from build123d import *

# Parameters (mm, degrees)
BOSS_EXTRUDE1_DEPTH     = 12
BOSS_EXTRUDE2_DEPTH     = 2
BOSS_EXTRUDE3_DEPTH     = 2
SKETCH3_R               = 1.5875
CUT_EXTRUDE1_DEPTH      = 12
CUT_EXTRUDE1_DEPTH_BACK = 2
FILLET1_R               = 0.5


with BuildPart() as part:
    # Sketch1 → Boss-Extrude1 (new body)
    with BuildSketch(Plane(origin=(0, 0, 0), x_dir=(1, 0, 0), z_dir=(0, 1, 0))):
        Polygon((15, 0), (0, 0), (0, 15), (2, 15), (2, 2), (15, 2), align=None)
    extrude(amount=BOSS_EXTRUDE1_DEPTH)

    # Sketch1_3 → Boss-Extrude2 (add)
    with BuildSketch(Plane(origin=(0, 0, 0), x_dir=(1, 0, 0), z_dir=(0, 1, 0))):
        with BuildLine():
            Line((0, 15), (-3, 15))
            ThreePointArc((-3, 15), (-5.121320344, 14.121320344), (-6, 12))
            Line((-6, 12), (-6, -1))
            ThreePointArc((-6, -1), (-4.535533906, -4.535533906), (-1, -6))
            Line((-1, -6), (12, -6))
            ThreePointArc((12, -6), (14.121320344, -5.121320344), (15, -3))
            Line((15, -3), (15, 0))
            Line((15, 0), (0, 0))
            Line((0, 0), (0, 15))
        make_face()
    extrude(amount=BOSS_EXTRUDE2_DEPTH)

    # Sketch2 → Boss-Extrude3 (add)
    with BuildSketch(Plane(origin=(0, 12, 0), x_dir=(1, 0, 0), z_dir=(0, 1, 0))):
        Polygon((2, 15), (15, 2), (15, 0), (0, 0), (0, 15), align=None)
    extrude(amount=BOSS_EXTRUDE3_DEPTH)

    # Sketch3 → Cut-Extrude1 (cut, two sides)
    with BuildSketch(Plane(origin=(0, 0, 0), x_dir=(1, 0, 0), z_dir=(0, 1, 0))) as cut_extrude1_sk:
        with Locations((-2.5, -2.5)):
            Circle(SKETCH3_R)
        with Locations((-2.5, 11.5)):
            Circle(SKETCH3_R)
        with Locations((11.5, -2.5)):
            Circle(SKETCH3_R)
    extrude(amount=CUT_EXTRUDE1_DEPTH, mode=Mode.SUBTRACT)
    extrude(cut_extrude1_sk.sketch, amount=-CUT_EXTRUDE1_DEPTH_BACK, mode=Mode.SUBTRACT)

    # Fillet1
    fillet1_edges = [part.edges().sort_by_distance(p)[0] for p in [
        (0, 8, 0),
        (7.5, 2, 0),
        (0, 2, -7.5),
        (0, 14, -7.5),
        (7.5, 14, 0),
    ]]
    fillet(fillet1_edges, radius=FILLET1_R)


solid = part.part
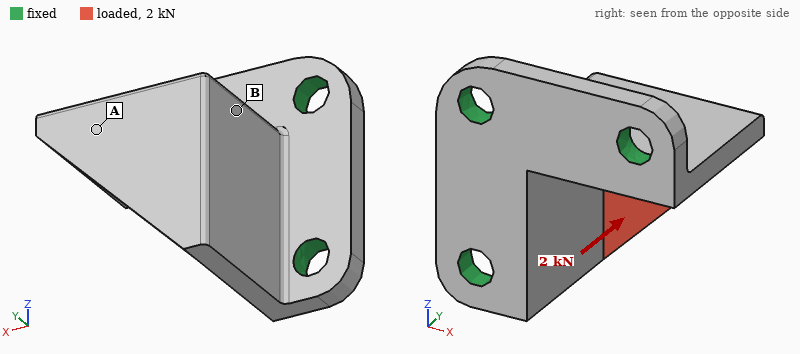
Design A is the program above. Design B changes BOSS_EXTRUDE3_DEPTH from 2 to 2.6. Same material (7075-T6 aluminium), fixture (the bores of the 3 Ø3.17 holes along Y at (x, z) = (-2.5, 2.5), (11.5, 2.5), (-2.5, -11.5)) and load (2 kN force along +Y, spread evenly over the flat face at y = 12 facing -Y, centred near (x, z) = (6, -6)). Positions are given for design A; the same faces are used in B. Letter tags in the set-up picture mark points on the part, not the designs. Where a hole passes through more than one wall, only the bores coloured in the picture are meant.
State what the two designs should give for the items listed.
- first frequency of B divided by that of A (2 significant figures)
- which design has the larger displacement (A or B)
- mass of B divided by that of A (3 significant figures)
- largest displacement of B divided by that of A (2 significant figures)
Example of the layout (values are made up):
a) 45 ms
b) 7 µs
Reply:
a) 0.96
b) A
c) 1.06
d) 0.79
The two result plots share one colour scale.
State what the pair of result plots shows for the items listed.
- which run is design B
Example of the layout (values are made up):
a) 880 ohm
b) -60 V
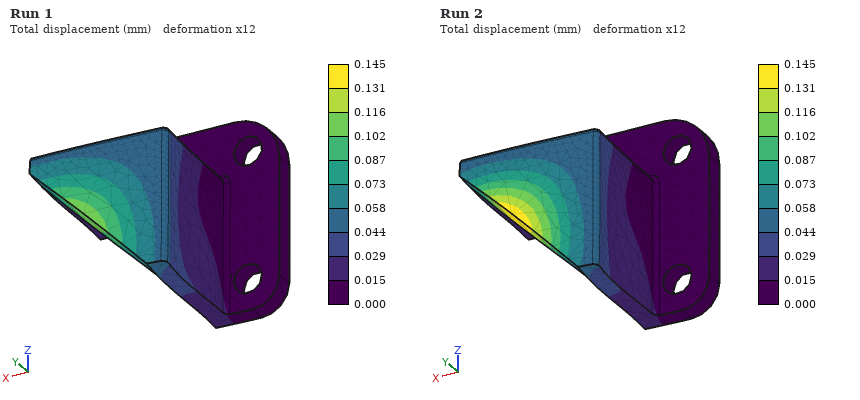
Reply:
a) Run 1
